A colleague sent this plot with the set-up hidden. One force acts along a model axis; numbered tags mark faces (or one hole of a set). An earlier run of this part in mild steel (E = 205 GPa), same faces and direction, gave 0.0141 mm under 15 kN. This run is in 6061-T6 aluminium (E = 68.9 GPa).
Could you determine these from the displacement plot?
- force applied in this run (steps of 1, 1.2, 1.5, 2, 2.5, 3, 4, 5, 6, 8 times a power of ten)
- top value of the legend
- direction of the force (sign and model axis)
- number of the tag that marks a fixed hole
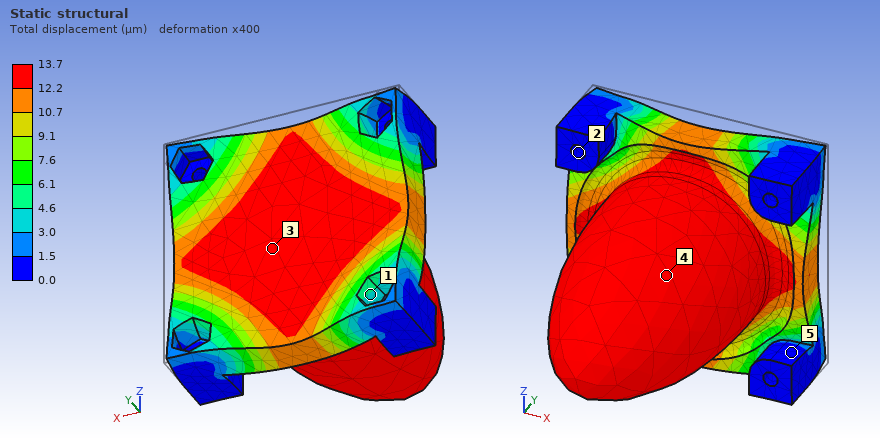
5 kN
13.7 µm
-Y
2
